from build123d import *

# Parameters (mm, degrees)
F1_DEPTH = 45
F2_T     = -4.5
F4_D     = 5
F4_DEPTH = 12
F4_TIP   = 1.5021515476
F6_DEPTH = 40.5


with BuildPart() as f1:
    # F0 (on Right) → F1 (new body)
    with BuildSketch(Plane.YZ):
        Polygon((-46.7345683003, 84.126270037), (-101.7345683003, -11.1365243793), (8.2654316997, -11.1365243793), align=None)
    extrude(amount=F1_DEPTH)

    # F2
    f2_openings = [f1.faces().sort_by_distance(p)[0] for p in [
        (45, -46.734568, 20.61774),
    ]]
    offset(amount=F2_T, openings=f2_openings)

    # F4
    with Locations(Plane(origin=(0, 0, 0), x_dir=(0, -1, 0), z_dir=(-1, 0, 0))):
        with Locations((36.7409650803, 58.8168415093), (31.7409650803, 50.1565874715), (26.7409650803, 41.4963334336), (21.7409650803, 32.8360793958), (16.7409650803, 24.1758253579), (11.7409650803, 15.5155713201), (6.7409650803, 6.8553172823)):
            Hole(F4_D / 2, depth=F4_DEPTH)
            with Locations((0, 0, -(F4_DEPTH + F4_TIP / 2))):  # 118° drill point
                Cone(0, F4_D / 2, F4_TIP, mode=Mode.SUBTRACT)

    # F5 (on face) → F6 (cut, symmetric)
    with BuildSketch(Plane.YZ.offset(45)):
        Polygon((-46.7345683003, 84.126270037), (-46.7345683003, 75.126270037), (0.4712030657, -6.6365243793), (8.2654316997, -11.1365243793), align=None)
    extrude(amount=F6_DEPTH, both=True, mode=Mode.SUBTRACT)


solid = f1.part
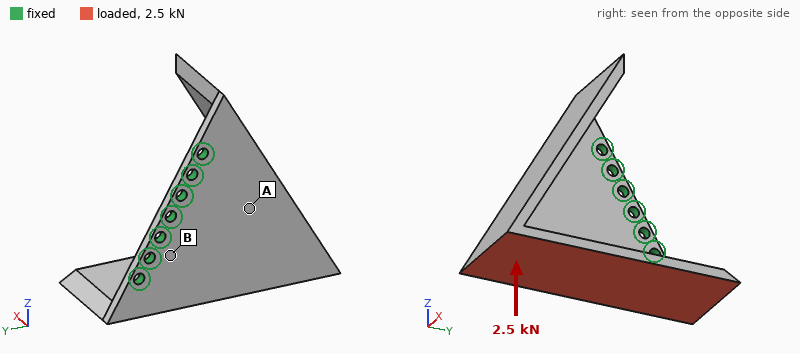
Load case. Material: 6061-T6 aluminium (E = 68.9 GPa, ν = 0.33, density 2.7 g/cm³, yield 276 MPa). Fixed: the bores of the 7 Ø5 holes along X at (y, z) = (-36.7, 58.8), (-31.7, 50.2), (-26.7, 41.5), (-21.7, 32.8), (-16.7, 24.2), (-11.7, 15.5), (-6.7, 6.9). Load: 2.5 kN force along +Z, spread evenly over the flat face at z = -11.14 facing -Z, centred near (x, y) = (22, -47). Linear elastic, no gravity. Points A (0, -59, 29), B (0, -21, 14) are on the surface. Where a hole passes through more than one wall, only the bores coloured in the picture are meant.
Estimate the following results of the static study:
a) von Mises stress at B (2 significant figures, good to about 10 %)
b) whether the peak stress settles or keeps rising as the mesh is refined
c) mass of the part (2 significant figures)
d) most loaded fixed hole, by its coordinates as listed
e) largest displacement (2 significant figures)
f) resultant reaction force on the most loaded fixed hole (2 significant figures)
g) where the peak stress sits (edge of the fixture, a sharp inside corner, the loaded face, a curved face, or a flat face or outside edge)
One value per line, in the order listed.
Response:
67 MPa
keeps rising
160 g
(-36.7, 58.8)
1.0 mm
1.3 kN
edge of the fixture
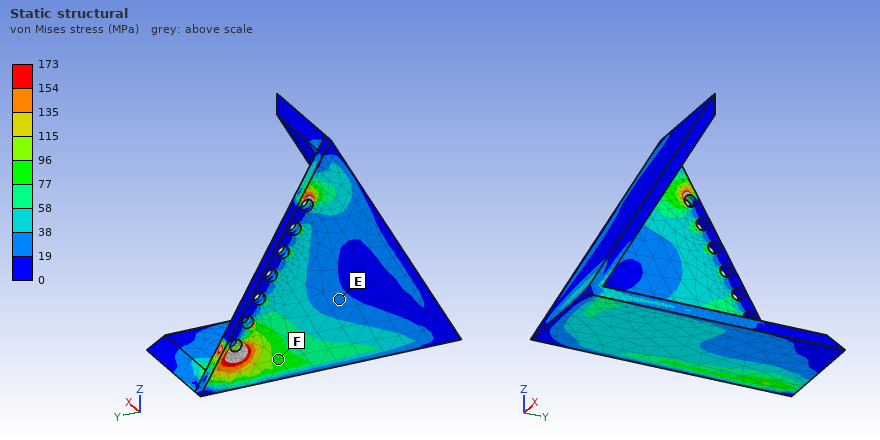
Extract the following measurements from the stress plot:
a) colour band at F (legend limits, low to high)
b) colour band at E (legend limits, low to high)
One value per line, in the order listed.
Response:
77 to 96 MPa
19 to 38 MPa
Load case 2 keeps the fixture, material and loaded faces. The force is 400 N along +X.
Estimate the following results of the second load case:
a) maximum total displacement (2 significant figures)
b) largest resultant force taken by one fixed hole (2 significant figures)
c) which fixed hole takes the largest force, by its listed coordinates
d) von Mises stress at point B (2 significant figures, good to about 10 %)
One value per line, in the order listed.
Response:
0.38 mm
200 N
(-6.7, 6.9)
39 MPa
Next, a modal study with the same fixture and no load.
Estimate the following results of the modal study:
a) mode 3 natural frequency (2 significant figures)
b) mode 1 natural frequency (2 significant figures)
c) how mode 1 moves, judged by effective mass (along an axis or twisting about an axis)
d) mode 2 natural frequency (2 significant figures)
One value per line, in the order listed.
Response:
1600 Hz
540 Hz
along X
1300 Hz
